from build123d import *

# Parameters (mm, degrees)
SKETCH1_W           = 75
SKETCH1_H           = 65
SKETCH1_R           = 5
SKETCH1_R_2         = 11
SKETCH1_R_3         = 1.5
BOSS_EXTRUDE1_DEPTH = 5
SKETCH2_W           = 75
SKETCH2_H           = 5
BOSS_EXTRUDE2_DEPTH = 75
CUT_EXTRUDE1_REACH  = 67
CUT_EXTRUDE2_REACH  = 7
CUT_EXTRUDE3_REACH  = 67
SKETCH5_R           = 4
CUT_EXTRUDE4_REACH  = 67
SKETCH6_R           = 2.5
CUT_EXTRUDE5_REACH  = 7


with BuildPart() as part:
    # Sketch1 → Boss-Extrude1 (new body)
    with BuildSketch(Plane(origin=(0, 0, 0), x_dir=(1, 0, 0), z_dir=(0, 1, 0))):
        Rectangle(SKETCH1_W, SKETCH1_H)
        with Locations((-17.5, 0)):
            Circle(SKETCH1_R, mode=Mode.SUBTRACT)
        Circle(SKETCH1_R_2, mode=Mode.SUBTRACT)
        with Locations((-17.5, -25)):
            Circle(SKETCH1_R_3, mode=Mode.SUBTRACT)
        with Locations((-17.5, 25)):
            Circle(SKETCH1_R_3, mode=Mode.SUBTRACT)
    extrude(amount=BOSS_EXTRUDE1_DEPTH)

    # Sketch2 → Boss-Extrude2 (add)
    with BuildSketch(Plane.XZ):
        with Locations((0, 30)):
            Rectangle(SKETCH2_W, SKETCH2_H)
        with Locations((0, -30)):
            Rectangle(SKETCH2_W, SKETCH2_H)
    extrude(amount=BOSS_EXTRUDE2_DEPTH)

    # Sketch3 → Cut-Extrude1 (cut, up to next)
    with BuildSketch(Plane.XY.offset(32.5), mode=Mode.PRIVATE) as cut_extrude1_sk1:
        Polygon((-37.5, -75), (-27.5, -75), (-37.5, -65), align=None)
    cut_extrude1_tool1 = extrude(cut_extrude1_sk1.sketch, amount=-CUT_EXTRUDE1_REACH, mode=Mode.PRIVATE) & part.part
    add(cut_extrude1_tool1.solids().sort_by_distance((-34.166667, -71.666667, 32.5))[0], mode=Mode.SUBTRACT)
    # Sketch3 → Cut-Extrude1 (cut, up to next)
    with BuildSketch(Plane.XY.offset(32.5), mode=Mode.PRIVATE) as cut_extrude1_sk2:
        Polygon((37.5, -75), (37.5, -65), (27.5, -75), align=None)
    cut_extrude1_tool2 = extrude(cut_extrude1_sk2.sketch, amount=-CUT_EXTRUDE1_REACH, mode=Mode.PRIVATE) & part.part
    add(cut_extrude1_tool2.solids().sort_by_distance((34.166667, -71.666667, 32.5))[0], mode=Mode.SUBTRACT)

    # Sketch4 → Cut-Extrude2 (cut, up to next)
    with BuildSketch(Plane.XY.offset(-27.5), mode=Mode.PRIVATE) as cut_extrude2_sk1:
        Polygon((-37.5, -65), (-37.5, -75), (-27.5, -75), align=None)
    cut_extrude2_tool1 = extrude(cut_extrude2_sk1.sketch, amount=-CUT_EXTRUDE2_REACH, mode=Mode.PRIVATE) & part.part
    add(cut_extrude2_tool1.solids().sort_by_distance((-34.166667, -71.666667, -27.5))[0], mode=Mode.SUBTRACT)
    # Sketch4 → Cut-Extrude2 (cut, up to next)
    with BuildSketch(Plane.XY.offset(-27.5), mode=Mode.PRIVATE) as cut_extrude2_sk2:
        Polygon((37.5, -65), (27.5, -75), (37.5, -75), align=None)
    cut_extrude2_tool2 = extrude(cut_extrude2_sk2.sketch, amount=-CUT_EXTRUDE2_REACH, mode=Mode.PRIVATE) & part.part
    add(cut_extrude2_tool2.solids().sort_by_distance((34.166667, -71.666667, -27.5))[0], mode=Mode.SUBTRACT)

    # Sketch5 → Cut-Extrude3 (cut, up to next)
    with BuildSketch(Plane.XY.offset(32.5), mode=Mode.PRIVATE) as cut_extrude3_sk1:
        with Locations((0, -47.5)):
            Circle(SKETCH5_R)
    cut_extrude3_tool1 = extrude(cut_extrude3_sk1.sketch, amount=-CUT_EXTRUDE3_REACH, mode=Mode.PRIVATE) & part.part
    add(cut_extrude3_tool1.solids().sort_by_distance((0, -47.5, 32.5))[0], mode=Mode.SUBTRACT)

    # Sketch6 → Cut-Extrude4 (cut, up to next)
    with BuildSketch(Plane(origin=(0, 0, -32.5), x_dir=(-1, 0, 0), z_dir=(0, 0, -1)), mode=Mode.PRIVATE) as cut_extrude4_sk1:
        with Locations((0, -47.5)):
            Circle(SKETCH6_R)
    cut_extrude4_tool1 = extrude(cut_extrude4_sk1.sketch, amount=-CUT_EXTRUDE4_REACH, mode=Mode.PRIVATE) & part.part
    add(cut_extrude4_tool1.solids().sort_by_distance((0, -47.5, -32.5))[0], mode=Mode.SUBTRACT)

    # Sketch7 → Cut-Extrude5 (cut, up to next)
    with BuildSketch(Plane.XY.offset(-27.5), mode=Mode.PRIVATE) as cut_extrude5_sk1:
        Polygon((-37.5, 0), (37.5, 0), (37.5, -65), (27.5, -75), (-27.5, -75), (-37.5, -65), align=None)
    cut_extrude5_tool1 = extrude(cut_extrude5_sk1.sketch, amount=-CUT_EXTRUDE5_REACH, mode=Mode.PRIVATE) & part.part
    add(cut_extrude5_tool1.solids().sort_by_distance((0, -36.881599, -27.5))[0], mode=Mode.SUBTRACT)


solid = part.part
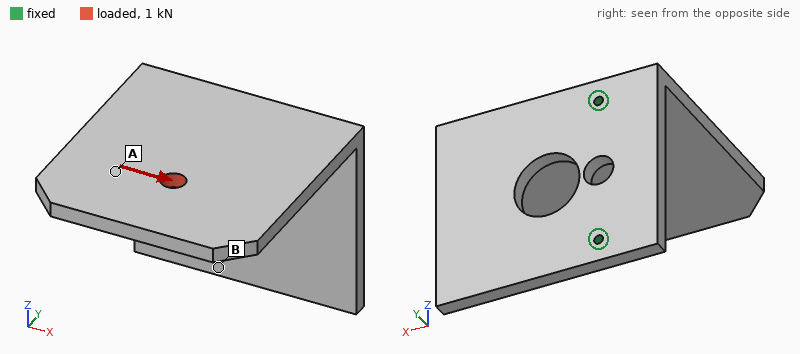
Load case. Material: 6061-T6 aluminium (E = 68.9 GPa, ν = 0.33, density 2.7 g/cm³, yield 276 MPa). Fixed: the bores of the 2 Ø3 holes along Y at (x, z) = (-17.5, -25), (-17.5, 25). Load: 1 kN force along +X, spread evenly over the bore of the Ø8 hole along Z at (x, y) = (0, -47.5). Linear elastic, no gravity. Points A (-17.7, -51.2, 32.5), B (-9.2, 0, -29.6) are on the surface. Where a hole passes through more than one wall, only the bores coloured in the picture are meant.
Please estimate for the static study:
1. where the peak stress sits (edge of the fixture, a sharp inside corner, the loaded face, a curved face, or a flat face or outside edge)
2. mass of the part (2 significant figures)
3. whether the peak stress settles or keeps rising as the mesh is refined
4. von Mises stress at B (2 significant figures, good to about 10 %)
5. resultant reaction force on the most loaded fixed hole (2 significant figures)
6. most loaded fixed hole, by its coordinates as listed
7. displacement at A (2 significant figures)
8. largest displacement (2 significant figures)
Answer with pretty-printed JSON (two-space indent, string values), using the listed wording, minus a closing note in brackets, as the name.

{
  "where the peak stress sits": "edge of the fixture",
  "mass of the part": "130 g",
  "whether the peak stress settles or keeps rising as the mesh is refined": "keeps rising",
  "von Mises stress at B": "57 MPa",
  "resultant reaction force on the most loaded fixed hole": "1.1 kN",
  "most loaded fixed hole, by its coordinates as listed": "(-17.5, 25)",
  "displacement at A": "0.64 mm",
  "largest displacement": "1.1 mm"
}
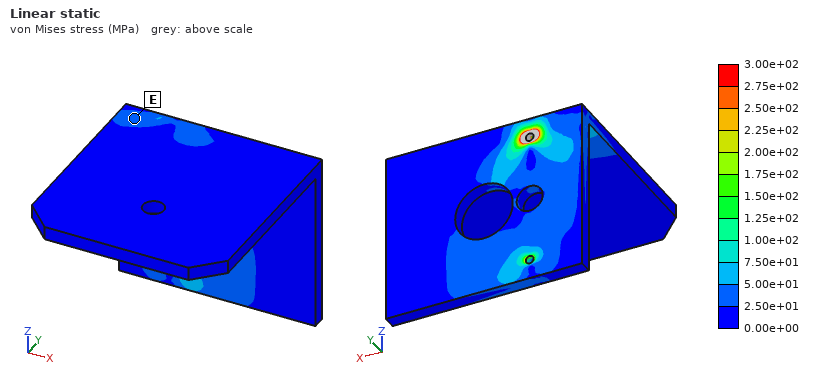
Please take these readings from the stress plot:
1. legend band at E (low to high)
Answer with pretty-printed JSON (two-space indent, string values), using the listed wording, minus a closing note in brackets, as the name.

{
  "legend band at E": "2.50e+01 to 5.00e+01 MPa"
}
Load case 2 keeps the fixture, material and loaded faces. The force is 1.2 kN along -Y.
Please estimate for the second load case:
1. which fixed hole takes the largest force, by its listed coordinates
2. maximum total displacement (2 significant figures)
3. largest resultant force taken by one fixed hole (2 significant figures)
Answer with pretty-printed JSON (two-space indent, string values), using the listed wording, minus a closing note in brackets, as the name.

{
  "which fixed hole takes the largest force, by its listed coordinates": "(-17.5, 25)",
  "maximum total displacement": "0.49 mm",
  "largest resultant force taken by one fixed hole": "1.2 kN"
}
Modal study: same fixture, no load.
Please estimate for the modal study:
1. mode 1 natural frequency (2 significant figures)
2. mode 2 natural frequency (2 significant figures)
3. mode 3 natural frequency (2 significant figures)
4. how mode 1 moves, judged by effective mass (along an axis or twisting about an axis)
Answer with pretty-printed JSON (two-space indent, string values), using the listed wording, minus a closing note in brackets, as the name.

{
  "mode 1 natural frequency": "540 Hz",
  "mode 2 natural frequency": "680 Hz",
  "mode 3 natural frequency": "1600 Hz",
  "how mode 1 moves, judged by effective mass": "along Z"
}
